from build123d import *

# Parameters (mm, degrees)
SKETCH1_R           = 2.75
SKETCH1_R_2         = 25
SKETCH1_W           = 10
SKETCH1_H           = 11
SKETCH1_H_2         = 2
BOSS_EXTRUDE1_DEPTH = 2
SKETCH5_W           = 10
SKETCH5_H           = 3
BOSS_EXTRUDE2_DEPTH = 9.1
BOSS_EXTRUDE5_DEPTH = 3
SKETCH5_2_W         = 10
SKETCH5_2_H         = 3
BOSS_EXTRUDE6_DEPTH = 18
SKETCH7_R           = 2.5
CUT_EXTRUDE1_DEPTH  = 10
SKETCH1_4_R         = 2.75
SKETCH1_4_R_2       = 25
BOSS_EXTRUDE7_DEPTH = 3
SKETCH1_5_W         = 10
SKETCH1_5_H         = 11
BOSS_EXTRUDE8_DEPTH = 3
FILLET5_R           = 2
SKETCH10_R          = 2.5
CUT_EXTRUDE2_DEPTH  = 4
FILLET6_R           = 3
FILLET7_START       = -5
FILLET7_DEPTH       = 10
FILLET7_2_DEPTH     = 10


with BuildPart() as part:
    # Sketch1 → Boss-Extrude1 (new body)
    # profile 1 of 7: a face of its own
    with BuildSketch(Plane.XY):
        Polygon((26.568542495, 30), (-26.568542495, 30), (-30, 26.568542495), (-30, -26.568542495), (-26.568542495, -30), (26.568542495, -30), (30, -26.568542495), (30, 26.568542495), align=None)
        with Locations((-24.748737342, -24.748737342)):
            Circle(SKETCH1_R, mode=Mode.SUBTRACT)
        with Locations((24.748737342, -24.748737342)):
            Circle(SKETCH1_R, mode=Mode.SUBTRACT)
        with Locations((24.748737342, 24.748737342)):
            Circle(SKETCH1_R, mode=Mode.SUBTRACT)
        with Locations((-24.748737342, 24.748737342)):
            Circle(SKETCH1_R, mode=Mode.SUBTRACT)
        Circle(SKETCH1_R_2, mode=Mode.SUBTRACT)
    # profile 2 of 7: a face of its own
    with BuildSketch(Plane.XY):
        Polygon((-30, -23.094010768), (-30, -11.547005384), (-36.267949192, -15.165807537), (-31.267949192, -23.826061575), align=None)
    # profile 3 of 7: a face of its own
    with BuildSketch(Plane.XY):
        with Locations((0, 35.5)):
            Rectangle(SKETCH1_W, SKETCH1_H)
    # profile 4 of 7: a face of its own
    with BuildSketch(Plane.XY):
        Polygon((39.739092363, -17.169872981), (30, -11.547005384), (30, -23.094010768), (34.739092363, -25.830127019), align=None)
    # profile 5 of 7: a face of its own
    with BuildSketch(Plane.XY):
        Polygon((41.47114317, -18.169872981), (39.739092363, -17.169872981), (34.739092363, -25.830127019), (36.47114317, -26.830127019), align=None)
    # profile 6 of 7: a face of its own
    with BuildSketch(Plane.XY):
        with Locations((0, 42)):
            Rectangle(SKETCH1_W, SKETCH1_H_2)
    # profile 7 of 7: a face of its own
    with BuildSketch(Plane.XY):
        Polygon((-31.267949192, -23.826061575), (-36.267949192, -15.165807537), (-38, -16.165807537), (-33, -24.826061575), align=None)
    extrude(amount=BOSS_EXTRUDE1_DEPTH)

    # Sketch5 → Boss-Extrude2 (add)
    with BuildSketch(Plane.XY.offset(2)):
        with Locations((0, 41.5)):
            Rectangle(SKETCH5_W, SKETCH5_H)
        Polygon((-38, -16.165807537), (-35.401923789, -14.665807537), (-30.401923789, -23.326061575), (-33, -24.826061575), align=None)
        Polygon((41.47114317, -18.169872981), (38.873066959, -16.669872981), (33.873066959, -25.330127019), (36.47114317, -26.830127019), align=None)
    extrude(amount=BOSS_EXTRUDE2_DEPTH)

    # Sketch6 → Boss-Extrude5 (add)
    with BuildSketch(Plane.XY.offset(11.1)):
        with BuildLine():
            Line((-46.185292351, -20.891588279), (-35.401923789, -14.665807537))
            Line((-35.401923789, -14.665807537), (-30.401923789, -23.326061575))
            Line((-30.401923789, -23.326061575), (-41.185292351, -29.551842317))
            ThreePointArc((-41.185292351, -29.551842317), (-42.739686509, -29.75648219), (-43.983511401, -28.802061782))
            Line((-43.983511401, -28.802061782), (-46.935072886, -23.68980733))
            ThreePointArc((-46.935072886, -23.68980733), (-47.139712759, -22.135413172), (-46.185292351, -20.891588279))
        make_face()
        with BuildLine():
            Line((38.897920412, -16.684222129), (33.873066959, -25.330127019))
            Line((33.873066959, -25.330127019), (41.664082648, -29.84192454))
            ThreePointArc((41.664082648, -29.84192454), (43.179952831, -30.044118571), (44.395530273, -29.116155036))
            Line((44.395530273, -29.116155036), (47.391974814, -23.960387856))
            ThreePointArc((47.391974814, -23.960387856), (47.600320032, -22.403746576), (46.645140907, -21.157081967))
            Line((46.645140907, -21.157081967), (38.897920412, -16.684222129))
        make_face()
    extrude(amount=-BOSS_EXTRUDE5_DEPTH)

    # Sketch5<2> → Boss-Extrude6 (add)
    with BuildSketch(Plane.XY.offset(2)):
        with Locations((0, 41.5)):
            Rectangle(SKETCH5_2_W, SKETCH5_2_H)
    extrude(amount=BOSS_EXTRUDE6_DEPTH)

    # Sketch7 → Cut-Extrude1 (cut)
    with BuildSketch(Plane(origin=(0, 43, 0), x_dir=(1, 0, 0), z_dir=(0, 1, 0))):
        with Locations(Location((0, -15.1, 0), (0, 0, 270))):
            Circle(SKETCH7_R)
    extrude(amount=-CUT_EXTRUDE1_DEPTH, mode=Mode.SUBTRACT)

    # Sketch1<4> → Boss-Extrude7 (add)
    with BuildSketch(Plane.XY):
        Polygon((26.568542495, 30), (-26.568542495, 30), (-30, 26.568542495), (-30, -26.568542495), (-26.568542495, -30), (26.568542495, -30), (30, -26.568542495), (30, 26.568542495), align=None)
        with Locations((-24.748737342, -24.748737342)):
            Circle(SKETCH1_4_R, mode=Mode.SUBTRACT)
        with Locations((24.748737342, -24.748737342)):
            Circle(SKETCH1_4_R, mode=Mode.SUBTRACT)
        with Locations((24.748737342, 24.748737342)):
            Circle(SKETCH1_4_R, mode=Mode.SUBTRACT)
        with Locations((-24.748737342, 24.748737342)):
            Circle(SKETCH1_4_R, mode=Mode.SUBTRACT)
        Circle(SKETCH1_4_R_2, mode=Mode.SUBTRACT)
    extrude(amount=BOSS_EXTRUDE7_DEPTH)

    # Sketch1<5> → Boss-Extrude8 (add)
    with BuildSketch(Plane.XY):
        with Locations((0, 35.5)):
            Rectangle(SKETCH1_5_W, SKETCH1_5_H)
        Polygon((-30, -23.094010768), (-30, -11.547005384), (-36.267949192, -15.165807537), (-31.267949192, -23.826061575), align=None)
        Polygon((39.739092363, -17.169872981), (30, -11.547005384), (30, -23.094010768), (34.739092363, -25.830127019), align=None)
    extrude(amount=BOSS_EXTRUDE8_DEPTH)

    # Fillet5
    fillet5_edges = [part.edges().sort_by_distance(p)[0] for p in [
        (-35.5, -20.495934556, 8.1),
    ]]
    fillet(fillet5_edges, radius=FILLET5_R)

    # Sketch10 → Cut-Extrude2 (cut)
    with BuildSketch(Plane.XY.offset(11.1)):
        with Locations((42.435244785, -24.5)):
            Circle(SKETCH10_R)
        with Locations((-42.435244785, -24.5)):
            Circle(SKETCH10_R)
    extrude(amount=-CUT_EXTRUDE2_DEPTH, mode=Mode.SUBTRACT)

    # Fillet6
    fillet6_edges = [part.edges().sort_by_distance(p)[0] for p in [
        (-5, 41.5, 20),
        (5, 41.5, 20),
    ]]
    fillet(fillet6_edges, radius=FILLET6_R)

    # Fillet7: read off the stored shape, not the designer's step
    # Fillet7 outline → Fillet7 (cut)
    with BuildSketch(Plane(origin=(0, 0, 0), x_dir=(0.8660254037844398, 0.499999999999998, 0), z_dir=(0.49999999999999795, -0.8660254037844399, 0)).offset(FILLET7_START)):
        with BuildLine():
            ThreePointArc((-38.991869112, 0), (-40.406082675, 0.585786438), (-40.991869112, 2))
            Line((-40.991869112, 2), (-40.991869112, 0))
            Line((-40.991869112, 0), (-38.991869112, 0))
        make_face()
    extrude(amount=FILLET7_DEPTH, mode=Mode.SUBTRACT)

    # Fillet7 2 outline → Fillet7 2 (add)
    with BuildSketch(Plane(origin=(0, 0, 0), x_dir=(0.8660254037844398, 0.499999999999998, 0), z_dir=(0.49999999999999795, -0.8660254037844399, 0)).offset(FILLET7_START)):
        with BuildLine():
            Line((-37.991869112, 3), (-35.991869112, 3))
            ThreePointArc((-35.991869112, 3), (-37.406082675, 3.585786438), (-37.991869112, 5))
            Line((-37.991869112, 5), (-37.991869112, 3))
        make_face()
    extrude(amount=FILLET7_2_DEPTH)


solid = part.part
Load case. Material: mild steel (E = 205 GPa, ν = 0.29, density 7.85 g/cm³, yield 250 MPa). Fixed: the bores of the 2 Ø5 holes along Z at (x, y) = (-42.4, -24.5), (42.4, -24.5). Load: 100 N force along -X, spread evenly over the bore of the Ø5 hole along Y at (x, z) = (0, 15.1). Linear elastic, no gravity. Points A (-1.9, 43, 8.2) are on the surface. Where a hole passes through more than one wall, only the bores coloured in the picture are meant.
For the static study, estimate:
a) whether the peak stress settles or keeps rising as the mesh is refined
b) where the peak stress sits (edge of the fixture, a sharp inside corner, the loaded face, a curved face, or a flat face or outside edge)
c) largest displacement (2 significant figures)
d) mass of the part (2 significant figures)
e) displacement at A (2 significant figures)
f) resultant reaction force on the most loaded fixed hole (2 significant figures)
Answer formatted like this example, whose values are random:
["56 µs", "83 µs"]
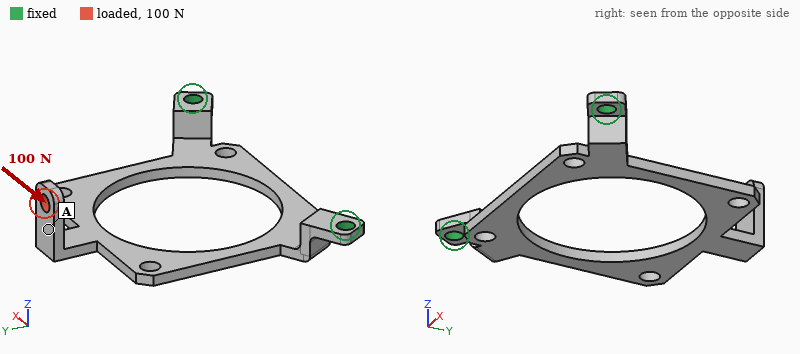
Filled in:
["keeps rising", "a sharp inside corner", "0.20 mm", "54 g", "0.094 mm", "100 N"]
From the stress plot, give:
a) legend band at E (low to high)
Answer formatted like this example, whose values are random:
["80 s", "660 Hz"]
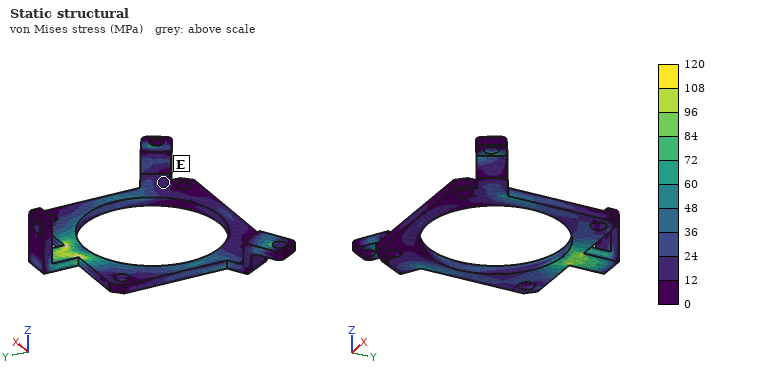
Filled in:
["12 to 24 MPa"]
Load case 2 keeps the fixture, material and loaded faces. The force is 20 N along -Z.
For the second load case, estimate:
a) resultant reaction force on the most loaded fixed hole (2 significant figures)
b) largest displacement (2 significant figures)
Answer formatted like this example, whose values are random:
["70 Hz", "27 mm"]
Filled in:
["33 N", "0.36 mm"]
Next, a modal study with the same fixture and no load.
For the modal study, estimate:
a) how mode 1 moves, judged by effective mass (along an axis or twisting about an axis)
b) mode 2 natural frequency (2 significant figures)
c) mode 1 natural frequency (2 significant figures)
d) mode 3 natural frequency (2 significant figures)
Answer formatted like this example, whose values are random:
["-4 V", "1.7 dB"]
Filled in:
["along Z", "1300 Hz", "370 Hz", "2000 Hz"]
